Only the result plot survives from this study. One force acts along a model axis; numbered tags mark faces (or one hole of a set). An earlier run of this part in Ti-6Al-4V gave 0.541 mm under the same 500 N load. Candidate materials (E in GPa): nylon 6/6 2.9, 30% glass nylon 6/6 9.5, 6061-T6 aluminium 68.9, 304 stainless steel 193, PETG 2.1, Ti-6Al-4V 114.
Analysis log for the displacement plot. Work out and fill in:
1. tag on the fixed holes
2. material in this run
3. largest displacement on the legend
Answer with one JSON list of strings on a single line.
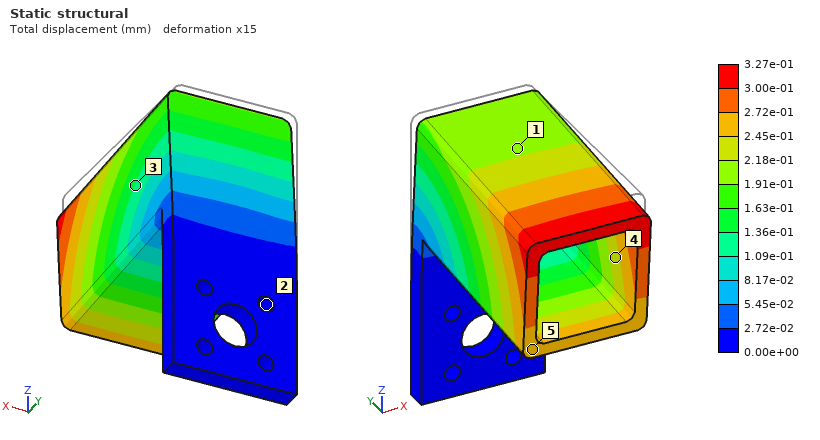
["2", "304 stainless steel", "3.27e-01 mm"]
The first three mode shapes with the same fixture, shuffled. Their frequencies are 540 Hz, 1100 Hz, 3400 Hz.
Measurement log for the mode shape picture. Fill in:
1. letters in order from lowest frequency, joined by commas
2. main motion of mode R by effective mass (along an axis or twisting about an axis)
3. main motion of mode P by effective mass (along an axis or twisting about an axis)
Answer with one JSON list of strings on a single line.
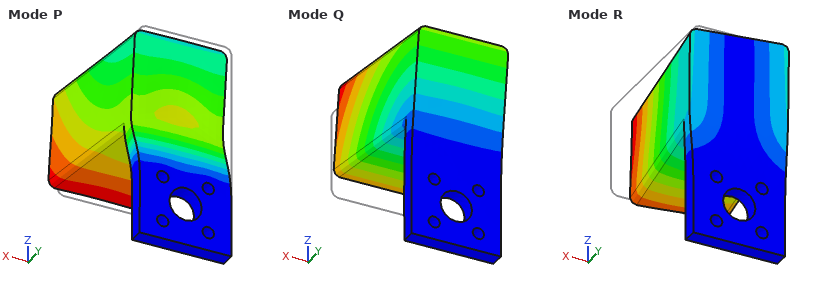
["Q, R, P", "along X", "along Y"]
